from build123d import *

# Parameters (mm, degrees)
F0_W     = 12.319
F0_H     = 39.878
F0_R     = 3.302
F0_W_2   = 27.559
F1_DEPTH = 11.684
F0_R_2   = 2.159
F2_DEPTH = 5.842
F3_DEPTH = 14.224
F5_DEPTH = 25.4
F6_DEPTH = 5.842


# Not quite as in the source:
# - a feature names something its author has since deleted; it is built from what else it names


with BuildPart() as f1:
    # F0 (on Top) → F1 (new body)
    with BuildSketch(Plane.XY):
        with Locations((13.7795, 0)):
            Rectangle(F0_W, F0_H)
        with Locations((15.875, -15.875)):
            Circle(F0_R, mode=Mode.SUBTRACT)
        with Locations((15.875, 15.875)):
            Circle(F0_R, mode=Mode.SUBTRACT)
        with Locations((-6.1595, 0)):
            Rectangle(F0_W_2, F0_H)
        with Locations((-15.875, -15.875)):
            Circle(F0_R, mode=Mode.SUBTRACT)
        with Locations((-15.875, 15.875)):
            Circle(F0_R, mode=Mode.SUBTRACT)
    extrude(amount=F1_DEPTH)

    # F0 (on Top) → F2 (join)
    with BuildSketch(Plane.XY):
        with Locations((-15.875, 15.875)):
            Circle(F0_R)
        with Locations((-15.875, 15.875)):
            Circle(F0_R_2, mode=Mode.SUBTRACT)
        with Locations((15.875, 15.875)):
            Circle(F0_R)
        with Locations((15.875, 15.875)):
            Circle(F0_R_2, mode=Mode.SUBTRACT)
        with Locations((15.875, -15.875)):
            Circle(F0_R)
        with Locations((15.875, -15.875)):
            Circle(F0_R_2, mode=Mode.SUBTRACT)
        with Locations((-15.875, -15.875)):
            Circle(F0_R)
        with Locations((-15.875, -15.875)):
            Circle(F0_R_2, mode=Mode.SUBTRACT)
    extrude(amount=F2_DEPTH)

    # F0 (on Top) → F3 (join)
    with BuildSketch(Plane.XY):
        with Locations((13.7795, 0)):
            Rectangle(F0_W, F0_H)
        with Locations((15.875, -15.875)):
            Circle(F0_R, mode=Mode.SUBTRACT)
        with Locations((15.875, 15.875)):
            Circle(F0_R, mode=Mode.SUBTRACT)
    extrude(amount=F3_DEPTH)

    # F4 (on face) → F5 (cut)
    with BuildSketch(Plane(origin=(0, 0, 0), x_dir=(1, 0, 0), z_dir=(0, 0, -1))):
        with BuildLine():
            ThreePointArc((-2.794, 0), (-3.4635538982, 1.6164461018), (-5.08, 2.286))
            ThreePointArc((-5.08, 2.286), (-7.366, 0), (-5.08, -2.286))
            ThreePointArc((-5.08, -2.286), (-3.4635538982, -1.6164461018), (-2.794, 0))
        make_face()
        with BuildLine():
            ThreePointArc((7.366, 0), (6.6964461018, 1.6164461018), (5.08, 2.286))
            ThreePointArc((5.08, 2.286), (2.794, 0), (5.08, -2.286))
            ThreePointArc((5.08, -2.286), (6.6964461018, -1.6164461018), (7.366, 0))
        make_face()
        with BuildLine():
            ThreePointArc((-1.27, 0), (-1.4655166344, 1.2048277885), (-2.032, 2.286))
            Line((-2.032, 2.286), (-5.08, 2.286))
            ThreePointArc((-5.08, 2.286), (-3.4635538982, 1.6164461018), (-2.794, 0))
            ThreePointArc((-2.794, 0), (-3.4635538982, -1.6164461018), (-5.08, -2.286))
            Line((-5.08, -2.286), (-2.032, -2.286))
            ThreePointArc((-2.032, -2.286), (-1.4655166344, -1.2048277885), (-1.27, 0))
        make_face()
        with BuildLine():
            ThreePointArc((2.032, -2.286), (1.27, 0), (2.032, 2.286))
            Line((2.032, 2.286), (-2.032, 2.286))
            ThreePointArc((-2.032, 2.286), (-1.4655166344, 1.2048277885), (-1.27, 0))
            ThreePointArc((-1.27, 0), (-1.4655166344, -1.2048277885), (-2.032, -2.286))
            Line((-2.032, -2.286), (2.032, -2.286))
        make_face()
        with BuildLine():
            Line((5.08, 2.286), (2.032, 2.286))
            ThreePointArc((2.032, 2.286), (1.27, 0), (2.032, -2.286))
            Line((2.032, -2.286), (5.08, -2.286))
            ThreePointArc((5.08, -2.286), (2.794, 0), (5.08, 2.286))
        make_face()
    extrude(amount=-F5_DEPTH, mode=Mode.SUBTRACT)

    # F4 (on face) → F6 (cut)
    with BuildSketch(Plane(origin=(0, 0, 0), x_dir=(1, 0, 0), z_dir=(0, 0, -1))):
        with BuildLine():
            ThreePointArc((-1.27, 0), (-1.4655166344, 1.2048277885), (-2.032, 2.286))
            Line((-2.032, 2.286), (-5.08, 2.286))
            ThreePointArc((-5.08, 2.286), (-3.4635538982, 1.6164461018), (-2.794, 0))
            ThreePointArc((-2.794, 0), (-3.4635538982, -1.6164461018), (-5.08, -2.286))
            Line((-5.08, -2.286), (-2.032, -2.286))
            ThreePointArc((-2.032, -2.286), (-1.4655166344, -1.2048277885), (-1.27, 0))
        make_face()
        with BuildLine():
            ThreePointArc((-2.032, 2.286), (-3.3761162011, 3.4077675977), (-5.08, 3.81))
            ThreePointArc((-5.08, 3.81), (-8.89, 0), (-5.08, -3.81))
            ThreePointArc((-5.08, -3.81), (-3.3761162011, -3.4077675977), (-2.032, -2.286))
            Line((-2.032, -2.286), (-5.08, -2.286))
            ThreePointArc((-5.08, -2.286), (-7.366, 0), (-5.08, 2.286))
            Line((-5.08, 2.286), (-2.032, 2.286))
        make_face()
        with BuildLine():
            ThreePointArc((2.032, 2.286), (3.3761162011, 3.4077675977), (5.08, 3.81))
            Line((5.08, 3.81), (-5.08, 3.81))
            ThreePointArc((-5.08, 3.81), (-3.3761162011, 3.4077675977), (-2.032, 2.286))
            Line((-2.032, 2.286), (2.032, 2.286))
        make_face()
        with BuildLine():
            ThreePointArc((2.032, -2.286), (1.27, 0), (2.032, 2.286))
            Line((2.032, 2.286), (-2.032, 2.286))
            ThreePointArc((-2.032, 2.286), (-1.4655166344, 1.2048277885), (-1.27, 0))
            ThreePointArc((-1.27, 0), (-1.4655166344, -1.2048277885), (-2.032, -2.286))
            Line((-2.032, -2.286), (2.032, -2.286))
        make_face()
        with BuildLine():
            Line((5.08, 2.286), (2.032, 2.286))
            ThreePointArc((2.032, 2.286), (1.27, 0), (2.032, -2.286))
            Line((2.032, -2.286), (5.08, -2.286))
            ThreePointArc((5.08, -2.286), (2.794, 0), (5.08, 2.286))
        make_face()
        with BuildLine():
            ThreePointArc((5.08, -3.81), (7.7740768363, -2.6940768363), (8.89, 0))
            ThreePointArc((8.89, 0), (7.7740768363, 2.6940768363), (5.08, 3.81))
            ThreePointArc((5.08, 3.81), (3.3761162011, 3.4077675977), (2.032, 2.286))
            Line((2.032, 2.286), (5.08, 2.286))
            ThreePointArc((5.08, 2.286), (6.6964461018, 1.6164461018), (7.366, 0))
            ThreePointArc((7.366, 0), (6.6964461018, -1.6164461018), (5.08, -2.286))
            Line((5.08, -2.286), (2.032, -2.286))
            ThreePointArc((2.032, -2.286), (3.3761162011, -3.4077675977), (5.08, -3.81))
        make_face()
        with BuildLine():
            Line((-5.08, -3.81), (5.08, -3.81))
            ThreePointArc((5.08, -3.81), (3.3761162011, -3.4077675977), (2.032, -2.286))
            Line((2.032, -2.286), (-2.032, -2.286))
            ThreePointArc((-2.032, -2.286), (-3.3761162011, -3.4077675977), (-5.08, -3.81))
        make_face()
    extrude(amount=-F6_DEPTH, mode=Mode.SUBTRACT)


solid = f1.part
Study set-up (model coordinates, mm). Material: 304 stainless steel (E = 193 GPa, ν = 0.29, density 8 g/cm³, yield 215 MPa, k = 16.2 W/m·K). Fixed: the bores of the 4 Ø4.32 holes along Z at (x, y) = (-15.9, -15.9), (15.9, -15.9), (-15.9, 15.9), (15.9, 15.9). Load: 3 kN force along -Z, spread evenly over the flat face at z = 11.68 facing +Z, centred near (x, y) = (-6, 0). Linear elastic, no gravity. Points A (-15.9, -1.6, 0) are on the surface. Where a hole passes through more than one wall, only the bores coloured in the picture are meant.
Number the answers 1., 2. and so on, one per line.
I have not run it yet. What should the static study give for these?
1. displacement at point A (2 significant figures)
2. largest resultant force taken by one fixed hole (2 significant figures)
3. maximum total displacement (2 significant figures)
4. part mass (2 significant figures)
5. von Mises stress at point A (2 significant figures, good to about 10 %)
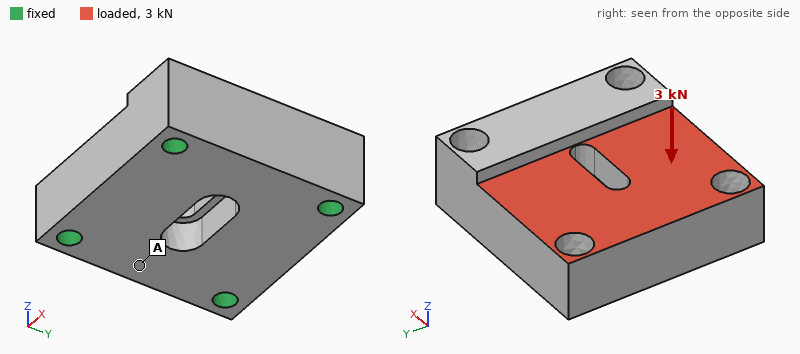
1. 1.5 µm
2. 1.1 kN
3. 2.1 µm
4. 140 g
5. 8.6 MPa
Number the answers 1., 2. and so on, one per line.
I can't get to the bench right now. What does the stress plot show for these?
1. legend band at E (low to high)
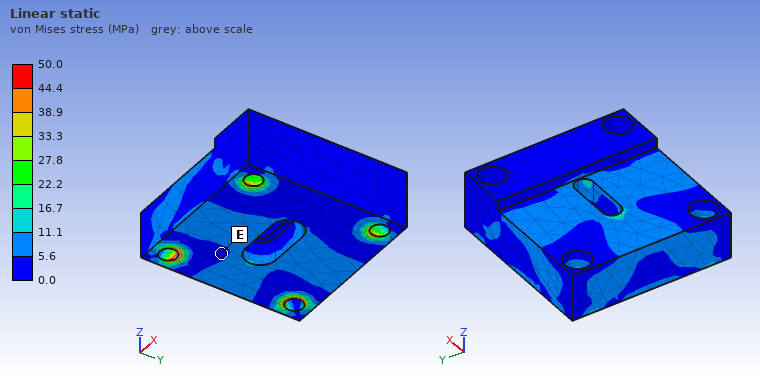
1. 0.0 to 5.6 MPa
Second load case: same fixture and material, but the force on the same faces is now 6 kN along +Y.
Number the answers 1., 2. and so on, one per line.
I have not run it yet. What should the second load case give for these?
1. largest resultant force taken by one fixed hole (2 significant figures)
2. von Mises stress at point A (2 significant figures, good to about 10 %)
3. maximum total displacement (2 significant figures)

1. 2.2 kN
2. 6.9 MPa
3. 3.4 µm
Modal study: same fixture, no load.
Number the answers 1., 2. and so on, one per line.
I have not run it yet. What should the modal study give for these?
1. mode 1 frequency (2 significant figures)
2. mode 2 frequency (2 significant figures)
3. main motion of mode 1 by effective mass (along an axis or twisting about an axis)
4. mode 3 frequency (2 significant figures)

1. 22 kHz
2. 31 kHz
3. along Z
4. 31 kHz
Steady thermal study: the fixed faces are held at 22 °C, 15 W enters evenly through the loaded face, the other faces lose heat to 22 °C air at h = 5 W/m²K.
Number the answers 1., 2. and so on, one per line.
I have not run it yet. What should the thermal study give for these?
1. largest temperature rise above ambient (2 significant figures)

1. 23 K
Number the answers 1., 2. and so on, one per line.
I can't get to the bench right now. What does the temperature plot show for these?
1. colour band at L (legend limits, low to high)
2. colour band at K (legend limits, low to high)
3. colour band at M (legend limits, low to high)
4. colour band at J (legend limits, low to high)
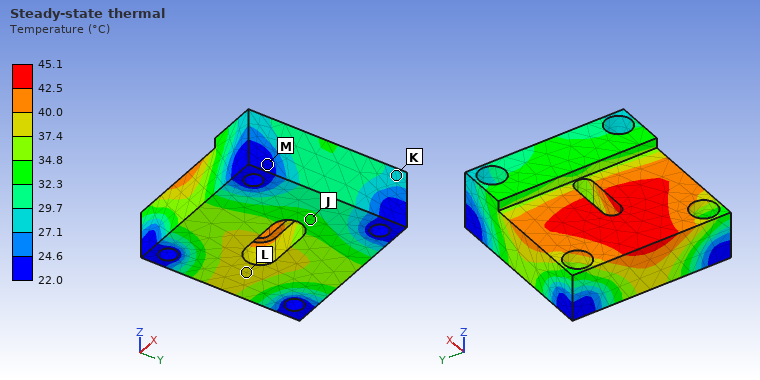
1. 37.4 to 40.0 °C
2. 27.1 to 29.7 °C
3. 22.0 to 24.6 °C
4. 32.3 to 34.8 °C
